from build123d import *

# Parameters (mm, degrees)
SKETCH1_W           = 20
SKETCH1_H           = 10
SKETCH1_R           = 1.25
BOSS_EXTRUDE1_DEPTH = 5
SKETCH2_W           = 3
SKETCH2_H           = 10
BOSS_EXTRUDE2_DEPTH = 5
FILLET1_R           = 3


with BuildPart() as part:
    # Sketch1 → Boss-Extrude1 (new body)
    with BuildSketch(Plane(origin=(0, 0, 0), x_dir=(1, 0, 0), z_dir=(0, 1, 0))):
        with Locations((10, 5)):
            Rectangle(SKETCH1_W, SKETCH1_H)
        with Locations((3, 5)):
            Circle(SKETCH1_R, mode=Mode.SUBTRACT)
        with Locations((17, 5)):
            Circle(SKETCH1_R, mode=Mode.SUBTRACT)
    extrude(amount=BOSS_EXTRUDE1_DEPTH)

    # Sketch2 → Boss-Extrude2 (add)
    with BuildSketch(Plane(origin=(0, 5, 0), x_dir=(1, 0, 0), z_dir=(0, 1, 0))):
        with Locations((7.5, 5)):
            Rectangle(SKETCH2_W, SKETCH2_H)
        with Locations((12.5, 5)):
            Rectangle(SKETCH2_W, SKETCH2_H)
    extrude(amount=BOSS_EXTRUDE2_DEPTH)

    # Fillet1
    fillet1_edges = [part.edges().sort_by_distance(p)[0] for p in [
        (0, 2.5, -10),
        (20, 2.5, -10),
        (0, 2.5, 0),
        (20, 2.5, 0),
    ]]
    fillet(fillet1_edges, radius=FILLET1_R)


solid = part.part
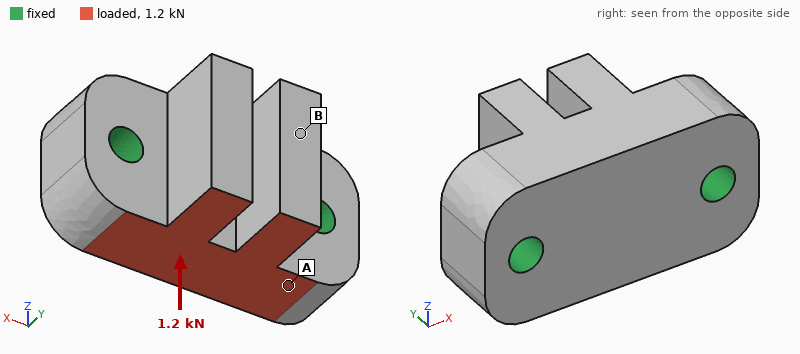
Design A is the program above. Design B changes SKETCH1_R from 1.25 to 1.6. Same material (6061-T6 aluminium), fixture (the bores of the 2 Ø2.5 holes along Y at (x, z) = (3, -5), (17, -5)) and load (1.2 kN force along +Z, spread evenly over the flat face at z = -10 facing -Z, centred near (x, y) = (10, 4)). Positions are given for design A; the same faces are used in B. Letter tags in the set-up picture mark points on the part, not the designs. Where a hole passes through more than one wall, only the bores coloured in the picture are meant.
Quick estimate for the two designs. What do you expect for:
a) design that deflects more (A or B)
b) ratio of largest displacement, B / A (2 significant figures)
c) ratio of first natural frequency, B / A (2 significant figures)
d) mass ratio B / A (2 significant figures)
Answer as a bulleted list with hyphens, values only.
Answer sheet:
- A
- 0.87
- 1.1
- 0.97
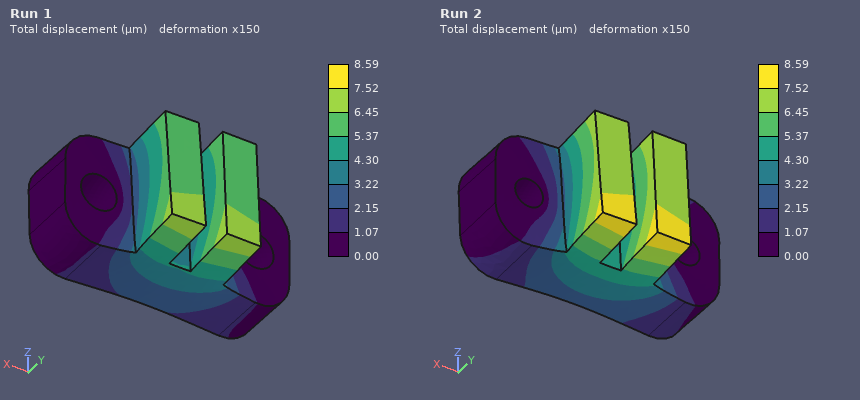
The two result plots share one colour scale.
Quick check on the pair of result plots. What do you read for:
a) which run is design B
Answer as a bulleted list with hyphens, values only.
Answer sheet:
- Run 1
